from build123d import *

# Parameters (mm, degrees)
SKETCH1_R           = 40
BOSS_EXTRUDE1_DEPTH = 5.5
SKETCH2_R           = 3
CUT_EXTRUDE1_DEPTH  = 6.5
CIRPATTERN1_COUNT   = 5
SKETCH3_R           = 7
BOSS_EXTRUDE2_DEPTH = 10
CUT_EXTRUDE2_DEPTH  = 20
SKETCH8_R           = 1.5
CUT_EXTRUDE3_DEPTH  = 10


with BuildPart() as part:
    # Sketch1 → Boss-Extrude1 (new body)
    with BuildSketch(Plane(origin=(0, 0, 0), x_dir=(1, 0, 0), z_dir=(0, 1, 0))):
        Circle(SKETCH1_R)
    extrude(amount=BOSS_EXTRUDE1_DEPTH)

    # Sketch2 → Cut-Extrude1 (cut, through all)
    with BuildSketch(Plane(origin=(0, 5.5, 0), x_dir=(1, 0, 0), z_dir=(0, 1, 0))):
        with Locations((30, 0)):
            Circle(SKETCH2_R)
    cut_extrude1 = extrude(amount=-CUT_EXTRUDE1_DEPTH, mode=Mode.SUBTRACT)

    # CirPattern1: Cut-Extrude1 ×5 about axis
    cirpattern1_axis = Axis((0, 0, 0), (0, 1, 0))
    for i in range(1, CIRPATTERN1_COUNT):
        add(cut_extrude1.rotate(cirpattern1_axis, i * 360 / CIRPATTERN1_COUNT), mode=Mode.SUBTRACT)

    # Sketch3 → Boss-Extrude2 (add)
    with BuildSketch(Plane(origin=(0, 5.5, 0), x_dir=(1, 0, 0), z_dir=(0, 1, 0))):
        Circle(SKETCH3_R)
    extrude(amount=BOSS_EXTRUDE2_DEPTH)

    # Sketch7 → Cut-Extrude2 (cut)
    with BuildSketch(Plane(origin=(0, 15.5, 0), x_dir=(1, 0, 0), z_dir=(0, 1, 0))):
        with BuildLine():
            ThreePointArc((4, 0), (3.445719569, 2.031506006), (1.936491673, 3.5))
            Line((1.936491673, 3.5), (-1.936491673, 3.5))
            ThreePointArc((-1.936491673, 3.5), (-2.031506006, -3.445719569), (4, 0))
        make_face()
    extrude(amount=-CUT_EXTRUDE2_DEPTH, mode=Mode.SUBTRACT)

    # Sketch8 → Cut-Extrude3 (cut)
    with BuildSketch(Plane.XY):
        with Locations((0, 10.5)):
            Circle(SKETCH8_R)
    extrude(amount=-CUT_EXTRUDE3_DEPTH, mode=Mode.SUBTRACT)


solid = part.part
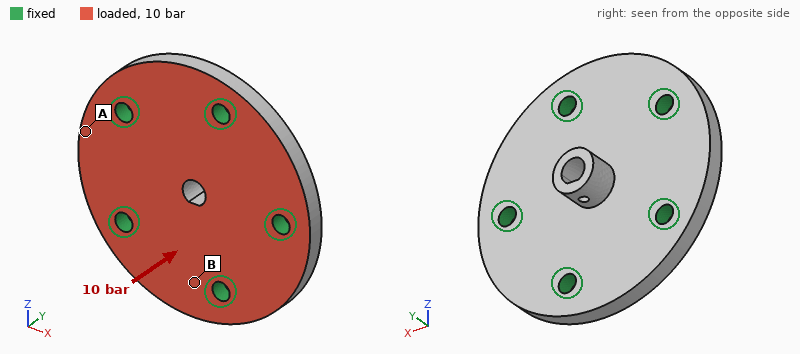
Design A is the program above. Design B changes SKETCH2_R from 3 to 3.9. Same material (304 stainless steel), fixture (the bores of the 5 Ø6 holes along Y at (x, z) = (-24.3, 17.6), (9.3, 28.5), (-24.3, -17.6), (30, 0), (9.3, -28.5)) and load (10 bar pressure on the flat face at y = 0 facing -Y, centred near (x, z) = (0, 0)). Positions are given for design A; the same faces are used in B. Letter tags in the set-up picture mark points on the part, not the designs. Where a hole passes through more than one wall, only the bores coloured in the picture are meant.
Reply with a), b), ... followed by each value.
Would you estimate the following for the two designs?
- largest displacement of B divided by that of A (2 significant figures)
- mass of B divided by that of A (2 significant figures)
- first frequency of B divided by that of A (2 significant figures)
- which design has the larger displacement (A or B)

a) 0.85
b) 0.98
c) 1.1
d) A
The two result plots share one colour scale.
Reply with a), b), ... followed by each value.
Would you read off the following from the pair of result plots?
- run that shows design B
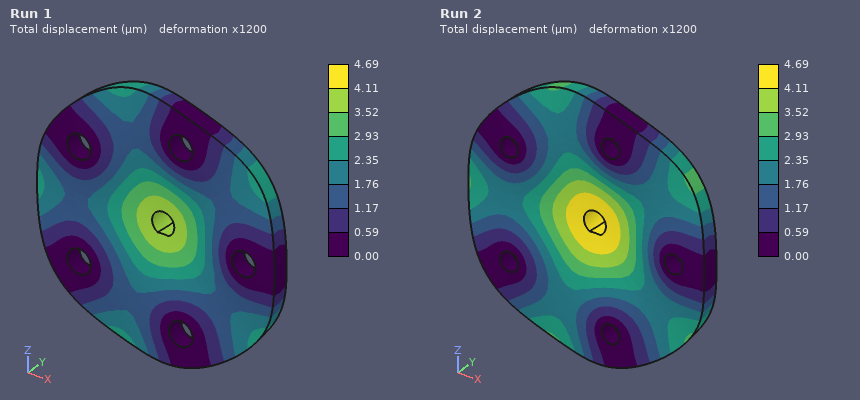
a) Run 1
